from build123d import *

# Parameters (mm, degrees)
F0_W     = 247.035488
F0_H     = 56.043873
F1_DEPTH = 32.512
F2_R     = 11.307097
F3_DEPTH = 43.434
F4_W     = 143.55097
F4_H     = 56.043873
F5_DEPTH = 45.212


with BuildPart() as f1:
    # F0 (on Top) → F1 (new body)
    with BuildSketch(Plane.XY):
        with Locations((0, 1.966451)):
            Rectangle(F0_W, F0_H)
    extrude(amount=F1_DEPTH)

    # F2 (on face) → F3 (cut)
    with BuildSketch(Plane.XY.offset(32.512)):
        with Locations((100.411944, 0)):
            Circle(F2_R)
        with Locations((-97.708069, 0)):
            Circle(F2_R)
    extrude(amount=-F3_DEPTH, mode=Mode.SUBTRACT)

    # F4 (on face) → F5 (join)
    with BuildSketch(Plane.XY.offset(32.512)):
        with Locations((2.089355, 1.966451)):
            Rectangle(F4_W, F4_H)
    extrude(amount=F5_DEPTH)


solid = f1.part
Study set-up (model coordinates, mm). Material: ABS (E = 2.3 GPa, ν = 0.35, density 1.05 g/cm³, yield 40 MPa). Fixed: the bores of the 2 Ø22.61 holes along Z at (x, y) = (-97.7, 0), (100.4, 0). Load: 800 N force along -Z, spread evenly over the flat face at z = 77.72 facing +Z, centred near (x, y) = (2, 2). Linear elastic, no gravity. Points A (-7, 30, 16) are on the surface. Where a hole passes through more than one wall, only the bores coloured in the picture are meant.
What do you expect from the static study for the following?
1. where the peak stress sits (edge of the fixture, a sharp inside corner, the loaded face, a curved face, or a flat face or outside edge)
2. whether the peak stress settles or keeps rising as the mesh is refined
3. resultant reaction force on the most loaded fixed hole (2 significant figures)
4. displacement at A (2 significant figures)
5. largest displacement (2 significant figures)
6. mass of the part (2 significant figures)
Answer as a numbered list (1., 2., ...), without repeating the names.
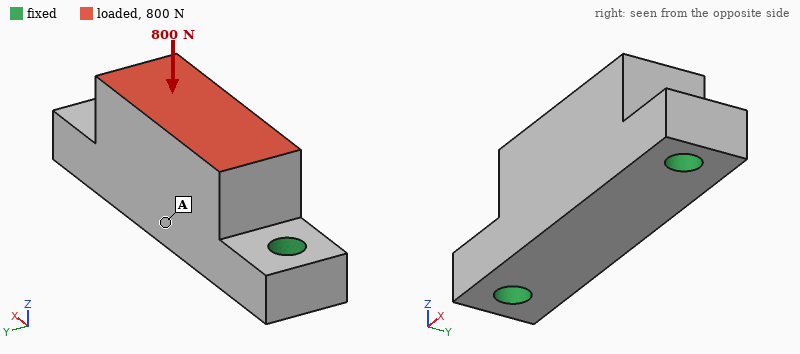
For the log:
1. edge of the fixture
2. keeps rising
3. 450 N
4. 22 µm
5. 23 µm
6. 830 g
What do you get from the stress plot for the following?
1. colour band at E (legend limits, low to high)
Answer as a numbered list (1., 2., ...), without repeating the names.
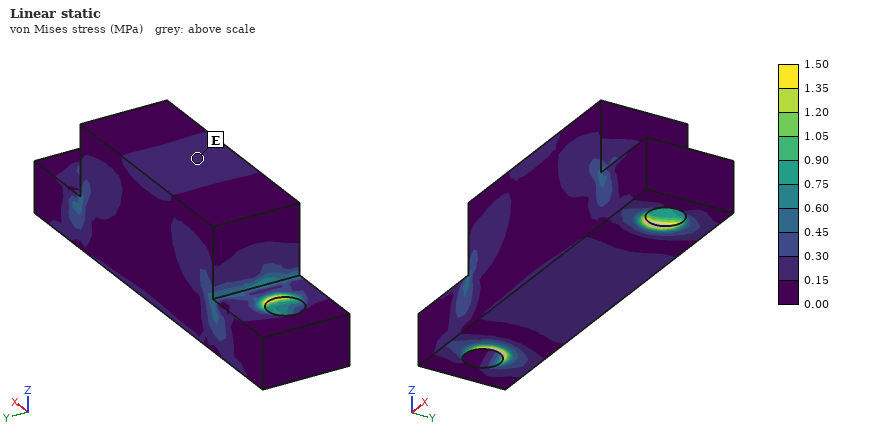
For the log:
1. 0.15 to 0.30 MPa
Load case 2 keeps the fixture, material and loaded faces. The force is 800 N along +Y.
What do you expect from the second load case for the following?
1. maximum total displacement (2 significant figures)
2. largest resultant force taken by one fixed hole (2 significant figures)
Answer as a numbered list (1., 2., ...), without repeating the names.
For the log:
1. 0.18 mm
2. 410 N
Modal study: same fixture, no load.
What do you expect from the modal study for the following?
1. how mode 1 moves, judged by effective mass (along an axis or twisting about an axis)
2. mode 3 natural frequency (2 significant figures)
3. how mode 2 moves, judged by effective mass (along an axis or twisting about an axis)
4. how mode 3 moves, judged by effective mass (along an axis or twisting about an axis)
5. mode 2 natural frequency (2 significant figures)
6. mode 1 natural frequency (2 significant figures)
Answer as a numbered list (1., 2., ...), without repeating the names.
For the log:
1. along Y
2. 1500 Hz
3. along Z
4. along Y
5. 1300 Hz
6. 730 Hz
